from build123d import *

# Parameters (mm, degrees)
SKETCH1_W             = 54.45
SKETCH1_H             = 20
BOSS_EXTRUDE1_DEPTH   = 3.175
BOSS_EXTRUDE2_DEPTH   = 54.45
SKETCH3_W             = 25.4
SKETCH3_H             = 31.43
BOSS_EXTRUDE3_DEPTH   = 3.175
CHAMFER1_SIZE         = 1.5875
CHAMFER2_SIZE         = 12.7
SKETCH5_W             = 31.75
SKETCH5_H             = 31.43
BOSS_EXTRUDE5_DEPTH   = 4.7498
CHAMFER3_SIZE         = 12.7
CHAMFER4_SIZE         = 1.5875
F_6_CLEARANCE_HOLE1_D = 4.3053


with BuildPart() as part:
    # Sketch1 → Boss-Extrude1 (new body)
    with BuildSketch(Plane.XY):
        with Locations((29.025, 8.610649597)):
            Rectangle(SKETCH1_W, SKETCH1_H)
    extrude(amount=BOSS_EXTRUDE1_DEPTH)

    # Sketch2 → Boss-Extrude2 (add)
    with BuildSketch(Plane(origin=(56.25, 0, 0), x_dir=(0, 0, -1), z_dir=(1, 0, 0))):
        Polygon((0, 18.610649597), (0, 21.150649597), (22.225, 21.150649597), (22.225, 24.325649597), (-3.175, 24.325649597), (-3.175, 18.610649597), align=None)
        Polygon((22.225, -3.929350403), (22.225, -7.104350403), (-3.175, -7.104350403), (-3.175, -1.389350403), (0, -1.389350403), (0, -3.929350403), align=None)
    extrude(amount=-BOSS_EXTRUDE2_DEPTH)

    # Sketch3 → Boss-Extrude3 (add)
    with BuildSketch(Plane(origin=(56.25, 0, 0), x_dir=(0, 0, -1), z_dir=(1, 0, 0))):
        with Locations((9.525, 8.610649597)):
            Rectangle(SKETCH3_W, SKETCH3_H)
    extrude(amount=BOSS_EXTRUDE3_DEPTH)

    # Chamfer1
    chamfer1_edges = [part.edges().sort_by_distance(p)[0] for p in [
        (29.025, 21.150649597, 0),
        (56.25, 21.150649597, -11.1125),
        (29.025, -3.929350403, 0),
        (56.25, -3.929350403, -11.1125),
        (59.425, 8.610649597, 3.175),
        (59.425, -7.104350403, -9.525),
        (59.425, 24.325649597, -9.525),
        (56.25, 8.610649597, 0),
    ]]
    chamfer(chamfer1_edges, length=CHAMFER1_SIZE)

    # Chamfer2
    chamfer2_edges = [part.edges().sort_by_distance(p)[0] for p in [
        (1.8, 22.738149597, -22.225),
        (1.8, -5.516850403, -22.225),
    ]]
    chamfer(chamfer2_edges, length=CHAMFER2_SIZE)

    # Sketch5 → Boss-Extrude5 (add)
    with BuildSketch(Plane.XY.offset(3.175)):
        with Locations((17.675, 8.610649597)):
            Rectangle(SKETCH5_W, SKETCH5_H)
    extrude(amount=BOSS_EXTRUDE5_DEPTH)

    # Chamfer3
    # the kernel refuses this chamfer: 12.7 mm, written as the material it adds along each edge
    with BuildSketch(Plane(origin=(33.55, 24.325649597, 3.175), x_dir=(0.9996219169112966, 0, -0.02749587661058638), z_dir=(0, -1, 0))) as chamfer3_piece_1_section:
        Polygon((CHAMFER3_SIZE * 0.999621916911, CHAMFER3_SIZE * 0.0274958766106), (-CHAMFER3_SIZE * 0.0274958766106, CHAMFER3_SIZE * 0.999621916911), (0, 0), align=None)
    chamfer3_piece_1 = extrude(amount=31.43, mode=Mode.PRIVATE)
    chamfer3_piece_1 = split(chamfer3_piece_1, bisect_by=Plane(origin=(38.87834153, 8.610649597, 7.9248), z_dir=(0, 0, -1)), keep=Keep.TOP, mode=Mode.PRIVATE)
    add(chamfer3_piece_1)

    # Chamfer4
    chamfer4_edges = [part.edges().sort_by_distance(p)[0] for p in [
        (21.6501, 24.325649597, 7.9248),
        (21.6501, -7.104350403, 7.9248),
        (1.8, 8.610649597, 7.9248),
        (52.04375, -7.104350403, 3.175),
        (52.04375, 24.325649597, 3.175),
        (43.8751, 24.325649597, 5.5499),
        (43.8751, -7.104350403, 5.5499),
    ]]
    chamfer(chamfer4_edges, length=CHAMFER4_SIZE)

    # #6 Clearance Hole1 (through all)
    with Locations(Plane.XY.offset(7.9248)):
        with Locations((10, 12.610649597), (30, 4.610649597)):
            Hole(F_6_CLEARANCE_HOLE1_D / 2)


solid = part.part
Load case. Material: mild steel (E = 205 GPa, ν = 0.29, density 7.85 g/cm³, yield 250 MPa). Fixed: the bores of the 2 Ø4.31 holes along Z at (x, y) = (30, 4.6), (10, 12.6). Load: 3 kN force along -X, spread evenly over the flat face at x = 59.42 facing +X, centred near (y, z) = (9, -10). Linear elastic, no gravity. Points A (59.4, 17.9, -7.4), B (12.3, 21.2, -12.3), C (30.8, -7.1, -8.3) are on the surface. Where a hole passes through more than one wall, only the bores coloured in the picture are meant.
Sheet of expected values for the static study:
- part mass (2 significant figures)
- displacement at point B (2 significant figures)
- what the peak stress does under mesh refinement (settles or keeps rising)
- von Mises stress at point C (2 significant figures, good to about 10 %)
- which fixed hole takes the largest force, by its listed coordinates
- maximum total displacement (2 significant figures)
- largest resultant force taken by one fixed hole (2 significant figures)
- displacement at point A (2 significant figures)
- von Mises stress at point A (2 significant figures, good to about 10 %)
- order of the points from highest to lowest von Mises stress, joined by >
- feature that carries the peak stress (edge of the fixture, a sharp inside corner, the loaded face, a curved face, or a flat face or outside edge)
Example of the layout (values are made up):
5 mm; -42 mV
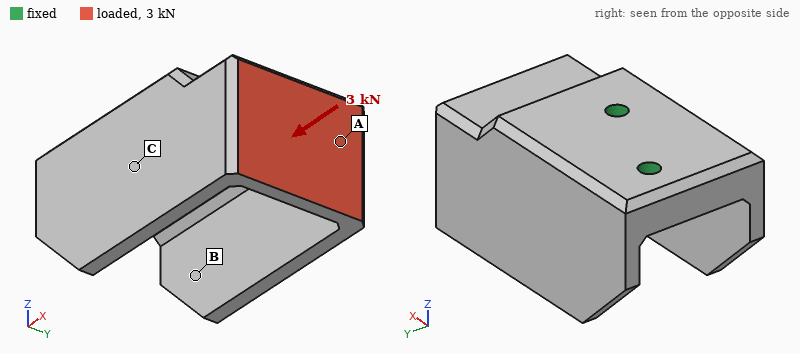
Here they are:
170 g; 7.1 µm; keeps rising; 27 MPa; (30, 4.6); 44 µm; 2.2 kN; 23 µm; 55 MPa; A > C > B; edge of the fixture
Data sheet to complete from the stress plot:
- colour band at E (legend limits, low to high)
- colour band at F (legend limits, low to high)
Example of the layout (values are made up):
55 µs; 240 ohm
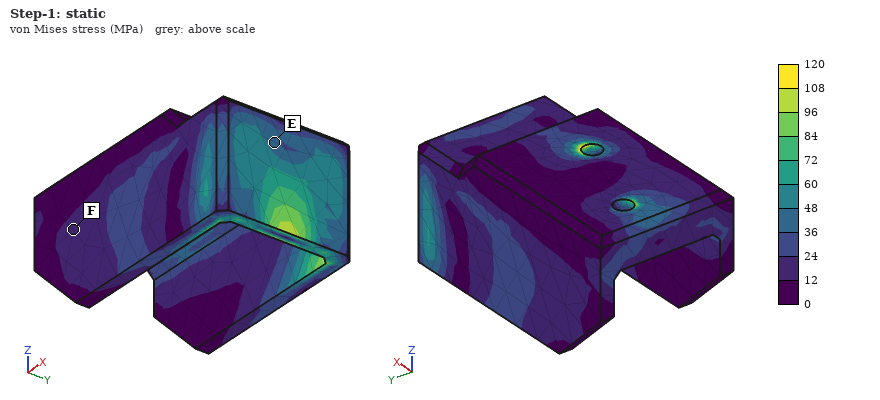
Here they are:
36 to 48 MPa; 12 to 24 MPa
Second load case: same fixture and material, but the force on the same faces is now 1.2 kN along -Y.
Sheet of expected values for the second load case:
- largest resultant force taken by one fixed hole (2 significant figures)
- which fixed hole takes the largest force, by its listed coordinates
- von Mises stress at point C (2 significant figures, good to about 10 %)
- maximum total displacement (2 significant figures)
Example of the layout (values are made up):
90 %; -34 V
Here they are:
2.4 kN; (30, 4.6); 18 MPa; 44 µm
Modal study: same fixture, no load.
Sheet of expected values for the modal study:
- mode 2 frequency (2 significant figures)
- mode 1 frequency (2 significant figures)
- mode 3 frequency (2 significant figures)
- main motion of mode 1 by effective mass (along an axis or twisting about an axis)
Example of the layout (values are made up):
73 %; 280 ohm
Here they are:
6100 Hz; 4100 Hz; 6200 Hz; along Y
